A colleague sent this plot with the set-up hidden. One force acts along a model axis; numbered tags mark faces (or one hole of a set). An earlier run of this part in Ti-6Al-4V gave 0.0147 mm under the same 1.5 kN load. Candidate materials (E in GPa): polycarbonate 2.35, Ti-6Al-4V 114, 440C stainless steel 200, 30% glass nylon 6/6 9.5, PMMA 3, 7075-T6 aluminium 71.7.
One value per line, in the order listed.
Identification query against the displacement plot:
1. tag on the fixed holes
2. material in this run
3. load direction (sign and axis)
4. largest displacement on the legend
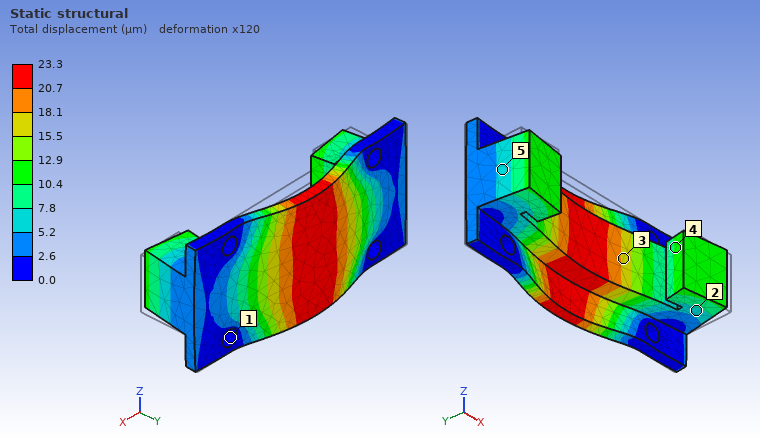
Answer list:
1
7075-T6 aluminium
+Y
23.3 µm
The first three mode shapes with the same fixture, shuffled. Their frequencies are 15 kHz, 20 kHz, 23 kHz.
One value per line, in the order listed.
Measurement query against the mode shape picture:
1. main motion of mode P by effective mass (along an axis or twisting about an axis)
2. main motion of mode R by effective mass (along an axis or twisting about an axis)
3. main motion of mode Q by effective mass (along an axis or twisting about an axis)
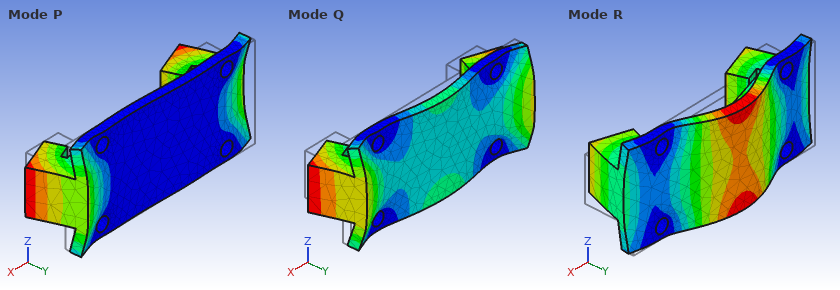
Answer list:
along X
along Y
along Y
